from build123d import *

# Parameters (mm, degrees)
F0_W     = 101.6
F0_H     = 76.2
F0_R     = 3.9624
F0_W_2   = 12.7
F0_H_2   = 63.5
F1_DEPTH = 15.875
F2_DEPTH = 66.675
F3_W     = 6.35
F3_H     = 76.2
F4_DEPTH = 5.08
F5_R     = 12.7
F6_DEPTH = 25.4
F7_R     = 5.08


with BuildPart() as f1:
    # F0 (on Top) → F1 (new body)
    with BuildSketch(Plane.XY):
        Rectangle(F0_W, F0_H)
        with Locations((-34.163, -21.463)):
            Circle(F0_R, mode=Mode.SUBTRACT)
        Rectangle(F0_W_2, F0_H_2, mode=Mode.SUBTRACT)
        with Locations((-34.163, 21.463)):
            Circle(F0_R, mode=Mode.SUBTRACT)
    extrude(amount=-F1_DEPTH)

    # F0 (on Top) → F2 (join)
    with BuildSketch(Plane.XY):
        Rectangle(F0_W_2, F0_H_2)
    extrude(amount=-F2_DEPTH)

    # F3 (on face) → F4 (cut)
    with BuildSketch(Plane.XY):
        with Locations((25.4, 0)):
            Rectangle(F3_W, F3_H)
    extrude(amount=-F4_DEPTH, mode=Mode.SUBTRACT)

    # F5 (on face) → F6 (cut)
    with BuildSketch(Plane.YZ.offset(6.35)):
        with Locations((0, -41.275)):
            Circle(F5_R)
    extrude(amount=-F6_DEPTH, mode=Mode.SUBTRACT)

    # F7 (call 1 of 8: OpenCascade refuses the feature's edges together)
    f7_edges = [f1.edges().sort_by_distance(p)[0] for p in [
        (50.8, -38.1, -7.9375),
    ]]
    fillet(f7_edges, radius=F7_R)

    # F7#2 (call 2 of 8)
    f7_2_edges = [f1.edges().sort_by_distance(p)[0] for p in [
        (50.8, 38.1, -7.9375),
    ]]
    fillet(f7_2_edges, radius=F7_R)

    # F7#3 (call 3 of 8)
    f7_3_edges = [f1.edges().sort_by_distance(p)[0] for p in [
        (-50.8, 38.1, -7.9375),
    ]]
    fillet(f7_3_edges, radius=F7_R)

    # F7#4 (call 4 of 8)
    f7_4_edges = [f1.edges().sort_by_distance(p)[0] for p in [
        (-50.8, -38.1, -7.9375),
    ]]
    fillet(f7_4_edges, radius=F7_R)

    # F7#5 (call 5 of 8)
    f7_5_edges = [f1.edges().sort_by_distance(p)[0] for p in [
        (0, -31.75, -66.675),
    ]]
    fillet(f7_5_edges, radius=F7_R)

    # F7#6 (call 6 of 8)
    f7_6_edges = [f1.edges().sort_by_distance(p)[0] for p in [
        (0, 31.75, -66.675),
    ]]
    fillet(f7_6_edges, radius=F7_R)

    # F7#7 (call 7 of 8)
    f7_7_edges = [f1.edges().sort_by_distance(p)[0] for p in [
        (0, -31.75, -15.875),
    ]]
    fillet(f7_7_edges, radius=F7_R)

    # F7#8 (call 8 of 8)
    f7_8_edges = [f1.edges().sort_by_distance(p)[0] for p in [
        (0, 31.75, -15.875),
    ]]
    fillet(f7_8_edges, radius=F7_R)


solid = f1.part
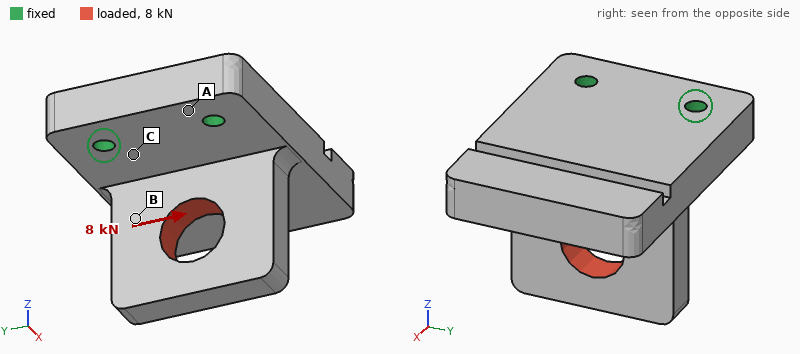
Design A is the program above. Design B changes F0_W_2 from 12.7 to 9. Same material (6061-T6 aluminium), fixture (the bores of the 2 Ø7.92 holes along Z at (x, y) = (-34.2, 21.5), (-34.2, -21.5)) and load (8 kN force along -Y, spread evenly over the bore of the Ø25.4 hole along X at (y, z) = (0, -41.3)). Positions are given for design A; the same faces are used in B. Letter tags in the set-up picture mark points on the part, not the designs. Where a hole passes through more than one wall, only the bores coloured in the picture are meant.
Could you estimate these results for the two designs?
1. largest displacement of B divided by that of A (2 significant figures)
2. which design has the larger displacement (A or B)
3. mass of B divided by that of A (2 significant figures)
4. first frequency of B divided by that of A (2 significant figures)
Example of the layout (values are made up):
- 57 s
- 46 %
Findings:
- 1.1
- B
- 0.93
- 1.0
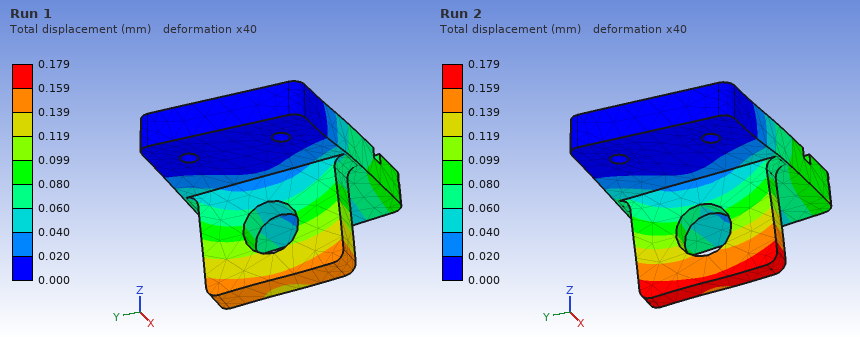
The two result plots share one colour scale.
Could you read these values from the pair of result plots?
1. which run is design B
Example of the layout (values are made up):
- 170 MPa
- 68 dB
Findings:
- Run 2
